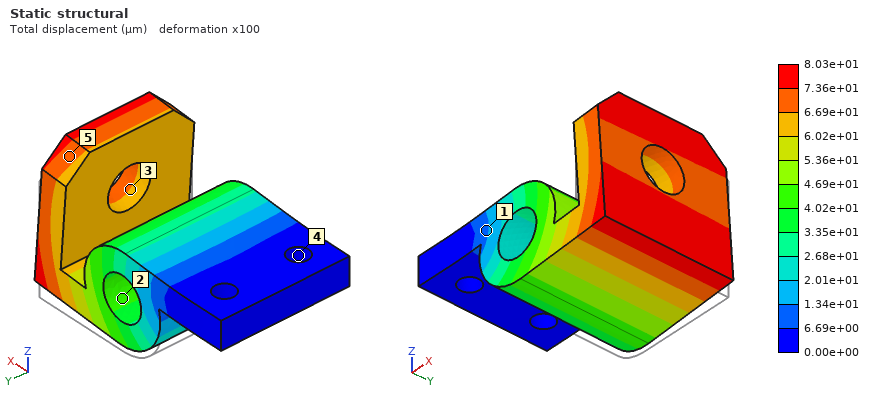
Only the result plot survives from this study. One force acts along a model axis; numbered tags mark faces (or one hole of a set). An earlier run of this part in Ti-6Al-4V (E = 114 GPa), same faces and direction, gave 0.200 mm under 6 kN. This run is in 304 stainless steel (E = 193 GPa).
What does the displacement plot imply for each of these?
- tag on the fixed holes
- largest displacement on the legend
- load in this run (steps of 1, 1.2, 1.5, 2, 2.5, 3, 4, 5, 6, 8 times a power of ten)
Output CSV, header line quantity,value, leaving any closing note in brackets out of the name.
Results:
quantity,value
tag on the fixed holes,4
largest displacement on the legend,8.03e+01 µm
load in this run,4 kN
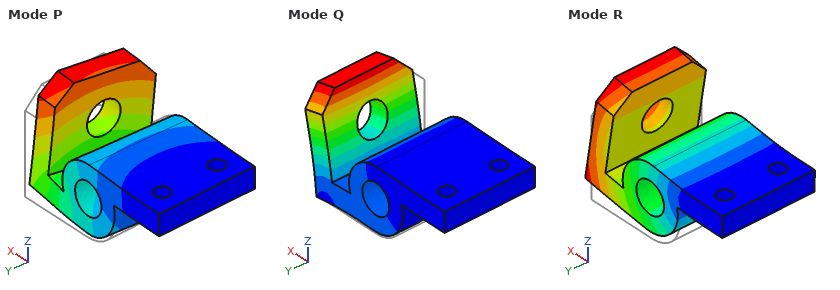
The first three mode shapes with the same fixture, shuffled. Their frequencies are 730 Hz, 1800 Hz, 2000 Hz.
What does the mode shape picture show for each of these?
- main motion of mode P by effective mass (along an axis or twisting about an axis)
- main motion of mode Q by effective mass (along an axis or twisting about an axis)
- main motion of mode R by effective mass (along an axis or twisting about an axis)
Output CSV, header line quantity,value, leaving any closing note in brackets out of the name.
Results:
quantity,value
main motion of mode P by effective mass,along Y
main motion of mode Q by effective mass,along X
main motion of mode R by effective mass,along Z
